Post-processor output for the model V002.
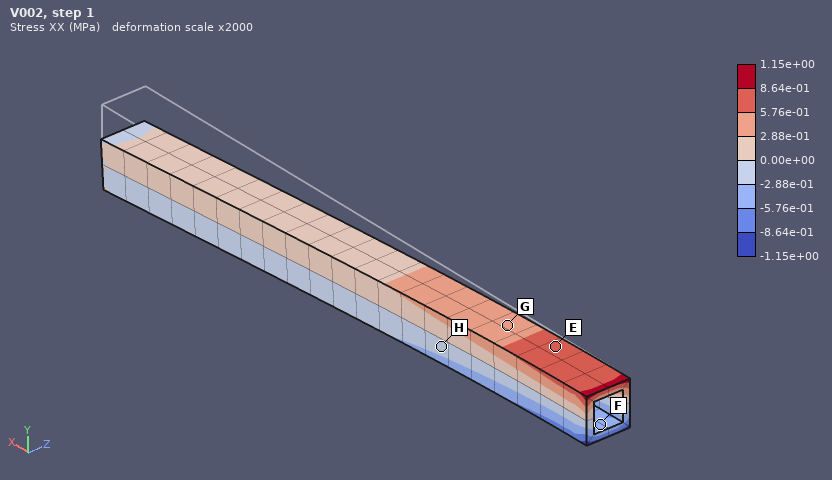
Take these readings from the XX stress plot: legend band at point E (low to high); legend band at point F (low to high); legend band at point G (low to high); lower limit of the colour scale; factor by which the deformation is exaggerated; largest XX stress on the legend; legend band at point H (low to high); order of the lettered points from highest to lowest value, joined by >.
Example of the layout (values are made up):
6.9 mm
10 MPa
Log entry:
5.76e-01 to 8.64e-01 MPa
-5.76e-01 to -2.88e-01 MPa
2.88e-01 to 5.76e-01 MPa
-1.15e+00 MPa
2000
1.15e+00 MPa
-2.88e-01 to 0.00e+00 MPa
E > G > H > F
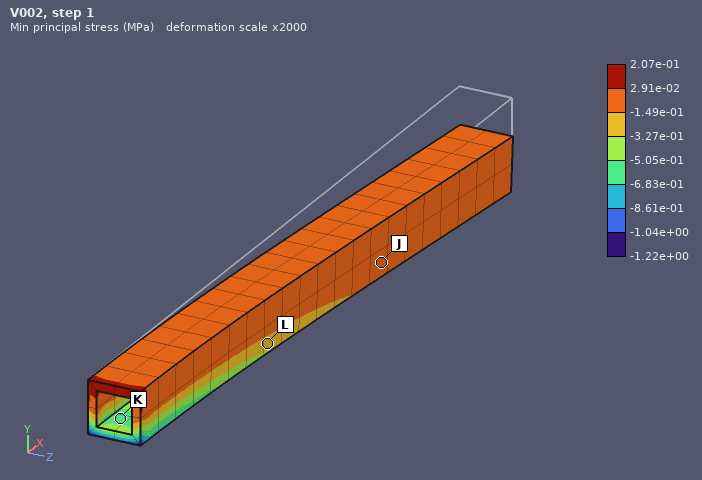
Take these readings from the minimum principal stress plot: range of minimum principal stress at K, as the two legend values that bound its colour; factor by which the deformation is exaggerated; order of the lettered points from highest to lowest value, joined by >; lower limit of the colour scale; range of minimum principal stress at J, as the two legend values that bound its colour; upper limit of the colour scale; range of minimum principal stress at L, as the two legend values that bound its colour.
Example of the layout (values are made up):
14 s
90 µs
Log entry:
-6.83e-01 to -5.05e-01 MPa
2000
J > L > K
-1.22e+00 MPa
-1.49e-01 to 2.91e-02 MPa
2.07e-01 MPa
-3.27e-01 to -1.49e-01 MPa
